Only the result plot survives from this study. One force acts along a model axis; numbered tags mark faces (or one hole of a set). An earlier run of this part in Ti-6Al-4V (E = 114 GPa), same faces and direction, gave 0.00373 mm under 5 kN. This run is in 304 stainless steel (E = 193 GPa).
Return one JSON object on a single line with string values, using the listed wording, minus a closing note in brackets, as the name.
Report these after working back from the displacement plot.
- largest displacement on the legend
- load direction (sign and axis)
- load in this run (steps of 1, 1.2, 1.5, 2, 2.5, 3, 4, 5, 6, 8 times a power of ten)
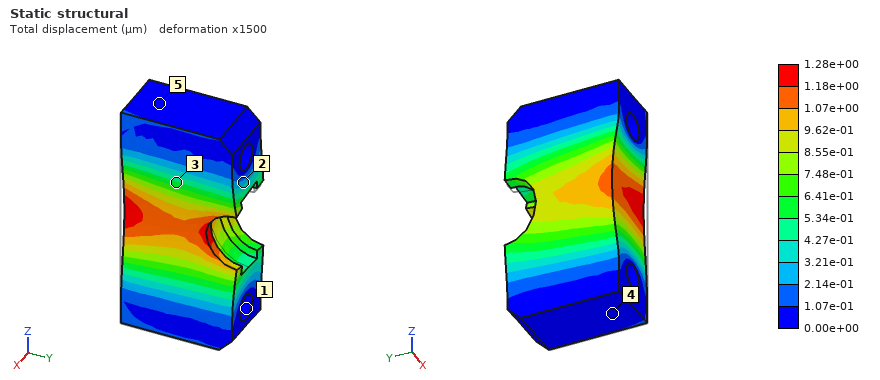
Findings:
{"largest displacement on the legend": "1.28e+00 µm", "load direction": "-X", "load in this run": "3 kN"}
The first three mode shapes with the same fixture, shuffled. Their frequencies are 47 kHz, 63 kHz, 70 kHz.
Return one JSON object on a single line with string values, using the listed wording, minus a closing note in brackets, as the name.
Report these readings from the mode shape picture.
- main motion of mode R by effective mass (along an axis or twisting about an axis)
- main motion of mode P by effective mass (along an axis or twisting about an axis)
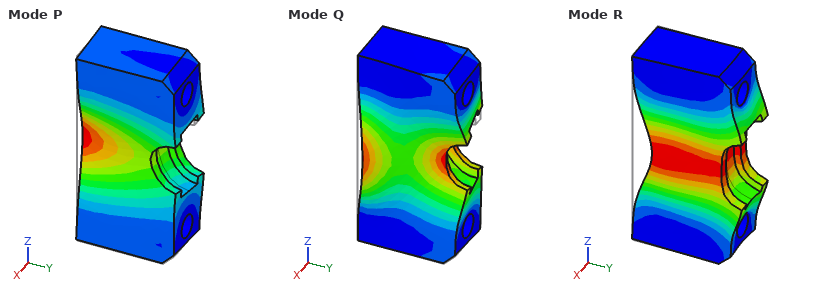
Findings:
{"main motion of mode R by effective mass": "along Y", "main motion of mode P by effective mass": "along X"}
